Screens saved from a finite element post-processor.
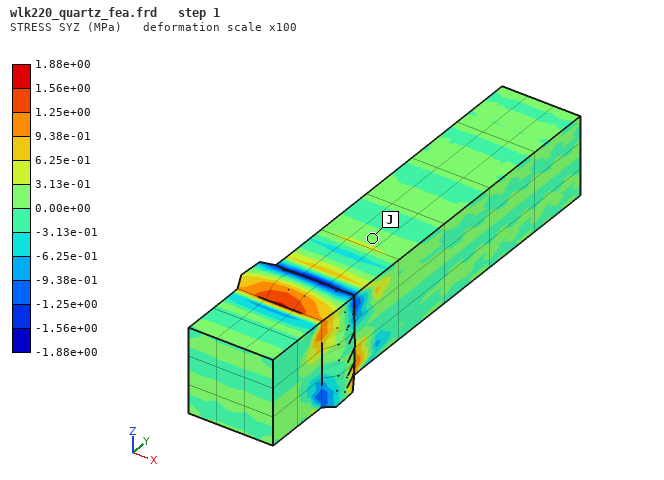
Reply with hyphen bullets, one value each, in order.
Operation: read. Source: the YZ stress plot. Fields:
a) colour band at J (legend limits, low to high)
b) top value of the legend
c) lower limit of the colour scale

- 0.00e+00 to 3.13e-01 MPa
- 1.88e+00 MPa
- -1.88e+00 MPa
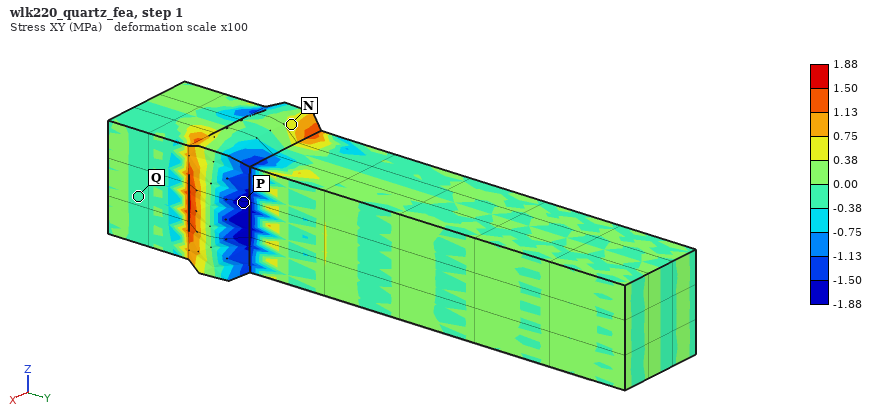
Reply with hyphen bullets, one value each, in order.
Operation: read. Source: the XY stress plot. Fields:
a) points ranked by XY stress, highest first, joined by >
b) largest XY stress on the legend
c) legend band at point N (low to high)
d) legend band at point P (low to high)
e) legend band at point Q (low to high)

- N > Q > P
- 1.88 MPa
- 0.38 to 0.75 MPa
- -1.88 to -1.50 MPa
- -0.38 to 0.00 MPa
